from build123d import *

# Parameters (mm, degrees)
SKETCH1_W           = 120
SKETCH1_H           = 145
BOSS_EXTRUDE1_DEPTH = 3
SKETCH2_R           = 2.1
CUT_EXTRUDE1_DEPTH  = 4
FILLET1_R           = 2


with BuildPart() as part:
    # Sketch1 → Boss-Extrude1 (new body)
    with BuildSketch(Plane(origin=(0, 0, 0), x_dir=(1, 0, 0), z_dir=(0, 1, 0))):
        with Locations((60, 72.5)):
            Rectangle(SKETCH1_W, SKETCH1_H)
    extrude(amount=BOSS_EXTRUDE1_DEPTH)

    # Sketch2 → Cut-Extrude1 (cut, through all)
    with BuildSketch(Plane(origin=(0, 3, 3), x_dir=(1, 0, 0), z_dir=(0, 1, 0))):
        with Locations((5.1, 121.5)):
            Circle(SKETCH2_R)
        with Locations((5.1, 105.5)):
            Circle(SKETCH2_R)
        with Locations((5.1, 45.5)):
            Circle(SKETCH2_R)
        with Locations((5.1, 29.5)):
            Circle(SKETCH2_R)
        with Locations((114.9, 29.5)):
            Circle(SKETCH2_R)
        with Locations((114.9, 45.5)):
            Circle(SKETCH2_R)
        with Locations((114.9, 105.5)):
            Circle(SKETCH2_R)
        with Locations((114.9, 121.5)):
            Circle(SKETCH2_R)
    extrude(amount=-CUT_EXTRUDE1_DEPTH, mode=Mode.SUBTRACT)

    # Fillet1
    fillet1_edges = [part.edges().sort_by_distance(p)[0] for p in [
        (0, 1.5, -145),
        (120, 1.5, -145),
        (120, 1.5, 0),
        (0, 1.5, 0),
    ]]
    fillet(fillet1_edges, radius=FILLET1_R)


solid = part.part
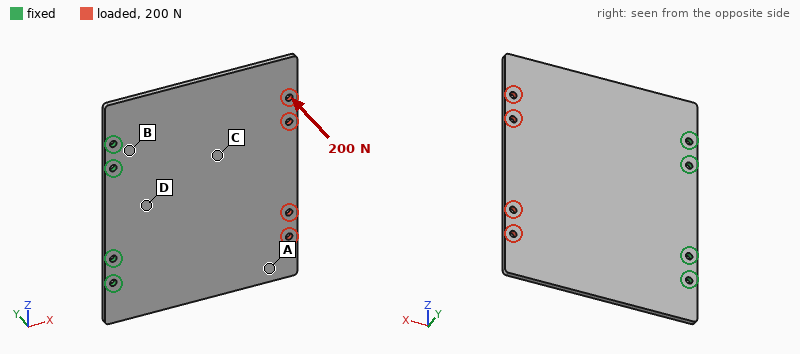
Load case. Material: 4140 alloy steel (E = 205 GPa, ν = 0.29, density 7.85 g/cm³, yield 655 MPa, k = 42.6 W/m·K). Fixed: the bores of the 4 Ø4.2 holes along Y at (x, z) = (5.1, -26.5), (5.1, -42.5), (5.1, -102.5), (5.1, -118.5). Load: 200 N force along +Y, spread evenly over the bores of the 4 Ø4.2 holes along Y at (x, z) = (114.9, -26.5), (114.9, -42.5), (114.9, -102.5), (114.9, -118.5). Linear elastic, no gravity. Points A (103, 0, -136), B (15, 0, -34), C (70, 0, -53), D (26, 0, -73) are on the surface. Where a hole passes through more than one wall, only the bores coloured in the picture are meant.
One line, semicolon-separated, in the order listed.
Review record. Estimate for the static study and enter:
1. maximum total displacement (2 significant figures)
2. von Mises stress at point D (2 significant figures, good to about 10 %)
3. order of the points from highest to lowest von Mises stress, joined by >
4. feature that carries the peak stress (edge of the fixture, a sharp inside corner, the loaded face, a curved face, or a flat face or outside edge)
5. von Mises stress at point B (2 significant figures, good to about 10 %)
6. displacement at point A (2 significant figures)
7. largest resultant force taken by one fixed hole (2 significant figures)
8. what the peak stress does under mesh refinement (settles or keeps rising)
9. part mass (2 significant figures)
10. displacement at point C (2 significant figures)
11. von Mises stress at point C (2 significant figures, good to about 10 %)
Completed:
1.6 mm; 68 MPa; B > D > C > A; edge of the fixture; 110 MPa; 1.2 mm; 94 N; keeps rising; 410 g; 0.65 mm; 38 MPa
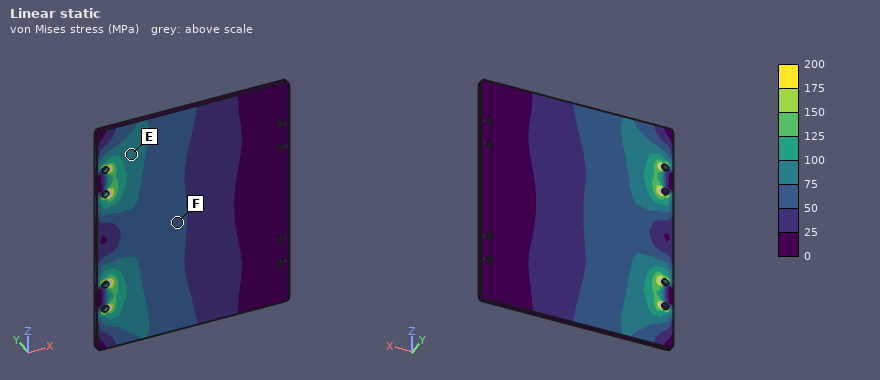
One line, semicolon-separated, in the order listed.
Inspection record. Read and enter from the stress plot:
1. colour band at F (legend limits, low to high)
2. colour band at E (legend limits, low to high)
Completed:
50 to 75 MPa; 75 to 100 MPa
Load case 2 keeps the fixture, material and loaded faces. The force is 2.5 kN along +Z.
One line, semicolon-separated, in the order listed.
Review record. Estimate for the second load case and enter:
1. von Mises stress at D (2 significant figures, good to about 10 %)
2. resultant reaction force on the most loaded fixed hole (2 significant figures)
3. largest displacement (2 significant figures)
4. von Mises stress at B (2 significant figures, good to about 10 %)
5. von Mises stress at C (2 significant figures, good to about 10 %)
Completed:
19 MPa; 2.4 kN; 31 µm; 33 MPa; 16 MPa
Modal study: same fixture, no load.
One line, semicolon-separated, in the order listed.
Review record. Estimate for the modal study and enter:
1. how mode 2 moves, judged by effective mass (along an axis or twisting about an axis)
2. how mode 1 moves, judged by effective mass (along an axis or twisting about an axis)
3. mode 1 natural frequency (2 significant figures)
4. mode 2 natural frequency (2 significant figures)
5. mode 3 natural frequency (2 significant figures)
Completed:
twisting about X; along Y; 180 Hz; 380 Hz; 950 Hz
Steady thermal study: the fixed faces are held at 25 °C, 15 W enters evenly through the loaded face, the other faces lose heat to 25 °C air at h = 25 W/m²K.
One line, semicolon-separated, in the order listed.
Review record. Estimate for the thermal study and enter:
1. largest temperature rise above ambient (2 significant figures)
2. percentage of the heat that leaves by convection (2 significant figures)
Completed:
49 K; 84 %
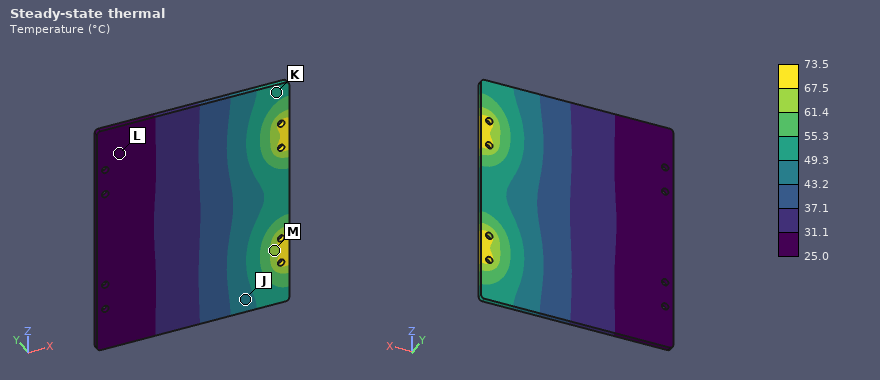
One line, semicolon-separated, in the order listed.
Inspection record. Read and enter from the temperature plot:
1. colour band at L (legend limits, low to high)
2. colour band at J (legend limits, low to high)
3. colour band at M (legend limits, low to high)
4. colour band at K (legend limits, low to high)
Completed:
25.0 to 31.1 °C; 43.2 to 49.3 °C; 61.4 to 67.5 °C; 49.3 to 55.3 °C
